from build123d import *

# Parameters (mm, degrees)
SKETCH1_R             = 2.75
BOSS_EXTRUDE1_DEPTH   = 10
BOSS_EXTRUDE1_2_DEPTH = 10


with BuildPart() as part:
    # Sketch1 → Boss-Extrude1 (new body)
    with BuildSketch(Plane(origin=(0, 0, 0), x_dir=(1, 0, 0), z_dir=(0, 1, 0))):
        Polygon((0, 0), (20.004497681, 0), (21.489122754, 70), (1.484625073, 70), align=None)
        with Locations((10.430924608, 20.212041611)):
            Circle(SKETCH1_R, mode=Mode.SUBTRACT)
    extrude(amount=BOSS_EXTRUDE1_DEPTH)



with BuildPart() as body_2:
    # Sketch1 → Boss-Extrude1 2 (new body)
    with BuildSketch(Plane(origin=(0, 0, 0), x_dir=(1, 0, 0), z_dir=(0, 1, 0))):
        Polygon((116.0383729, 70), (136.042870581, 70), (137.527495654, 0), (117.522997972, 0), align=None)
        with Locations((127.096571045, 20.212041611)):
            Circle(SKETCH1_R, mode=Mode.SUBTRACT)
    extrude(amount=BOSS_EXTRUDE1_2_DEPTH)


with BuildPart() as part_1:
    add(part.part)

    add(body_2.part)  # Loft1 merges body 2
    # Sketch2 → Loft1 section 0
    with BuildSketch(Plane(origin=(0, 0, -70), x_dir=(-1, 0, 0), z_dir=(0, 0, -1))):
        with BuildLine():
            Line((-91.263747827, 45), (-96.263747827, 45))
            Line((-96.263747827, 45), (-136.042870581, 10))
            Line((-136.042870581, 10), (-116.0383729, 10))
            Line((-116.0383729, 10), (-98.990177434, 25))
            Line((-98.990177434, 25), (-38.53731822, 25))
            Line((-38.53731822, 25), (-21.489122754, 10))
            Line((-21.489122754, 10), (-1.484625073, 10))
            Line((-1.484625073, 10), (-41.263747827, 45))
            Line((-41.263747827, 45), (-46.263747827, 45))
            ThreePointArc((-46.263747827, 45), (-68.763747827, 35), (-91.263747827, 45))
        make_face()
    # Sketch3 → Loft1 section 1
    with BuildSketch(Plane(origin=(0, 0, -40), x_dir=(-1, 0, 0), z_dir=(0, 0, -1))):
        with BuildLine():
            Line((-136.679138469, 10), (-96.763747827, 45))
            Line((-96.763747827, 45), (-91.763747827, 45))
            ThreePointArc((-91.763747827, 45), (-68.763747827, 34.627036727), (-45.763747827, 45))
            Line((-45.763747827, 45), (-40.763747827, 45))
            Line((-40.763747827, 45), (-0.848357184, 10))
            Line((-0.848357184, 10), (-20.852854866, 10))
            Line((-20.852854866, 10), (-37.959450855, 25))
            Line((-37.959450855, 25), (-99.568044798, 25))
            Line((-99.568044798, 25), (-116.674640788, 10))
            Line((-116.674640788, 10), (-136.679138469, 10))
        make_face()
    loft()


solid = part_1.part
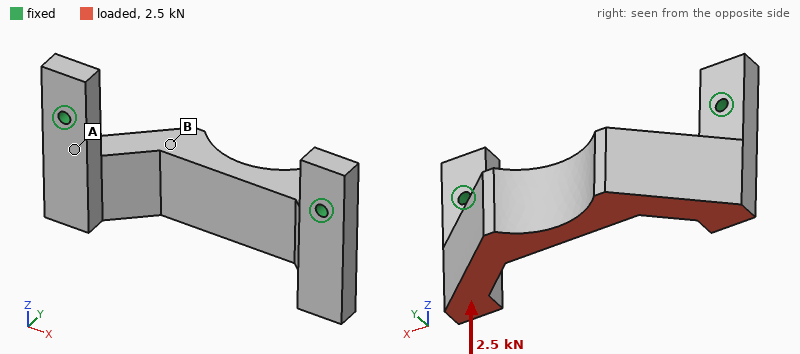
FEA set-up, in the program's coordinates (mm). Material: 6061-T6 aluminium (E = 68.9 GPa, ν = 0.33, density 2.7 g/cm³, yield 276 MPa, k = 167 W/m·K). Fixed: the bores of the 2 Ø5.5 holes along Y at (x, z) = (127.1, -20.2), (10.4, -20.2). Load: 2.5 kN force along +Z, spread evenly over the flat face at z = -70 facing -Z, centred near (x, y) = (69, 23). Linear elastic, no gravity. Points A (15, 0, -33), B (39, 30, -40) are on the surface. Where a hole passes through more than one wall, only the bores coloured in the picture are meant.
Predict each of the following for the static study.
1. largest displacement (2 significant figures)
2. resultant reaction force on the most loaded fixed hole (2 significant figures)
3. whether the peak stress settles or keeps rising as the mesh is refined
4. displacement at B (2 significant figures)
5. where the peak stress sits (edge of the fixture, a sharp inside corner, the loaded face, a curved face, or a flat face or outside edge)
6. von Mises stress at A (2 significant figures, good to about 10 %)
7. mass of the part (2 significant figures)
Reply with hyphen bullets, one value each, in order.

- 0.31 mm
- 1.3 kN
- keeps rising
- 0.15 mm
- edge of the fixture
- 58 MPa
- 220 g
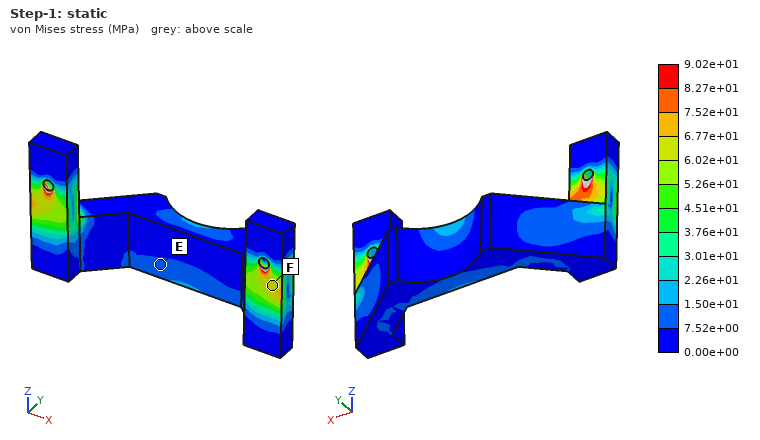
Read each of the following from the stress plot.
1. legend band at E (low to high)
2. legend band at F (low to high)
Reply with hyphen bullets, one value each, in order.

- 7.52e+00 to 1.50e+01 MPa
- 6.02e+01 to 6.77e+01 MPa
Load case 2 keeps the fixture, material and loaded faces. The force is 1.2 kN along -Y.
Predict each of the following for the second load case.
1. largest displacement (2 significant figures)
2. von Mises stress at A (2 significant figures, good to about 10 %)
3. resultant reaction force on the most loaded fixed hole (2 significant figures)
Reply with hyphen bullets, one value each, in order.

- 0.30 mm
- 64 MPa
- 650 N
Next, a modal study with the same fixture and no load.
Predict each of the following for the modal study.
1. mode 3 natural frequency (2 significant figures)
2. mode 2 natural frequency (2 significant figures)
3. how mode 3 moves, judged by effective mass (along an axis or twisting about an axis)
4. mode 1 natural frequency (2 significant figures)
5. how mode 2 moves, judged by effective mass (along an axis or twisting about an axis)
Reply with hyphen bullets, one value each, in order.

- 3100 Hz
- 2700 Hz
- along X
- 1000 Hz
- along X
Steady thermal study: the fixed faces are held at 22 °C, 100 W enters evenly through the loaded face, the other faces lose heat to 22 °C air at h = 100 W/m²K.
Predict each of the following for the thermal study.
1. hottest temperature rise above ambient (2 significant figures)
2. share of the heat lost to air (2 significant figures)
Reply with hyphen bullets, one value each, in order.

- 39 K
- 41 %
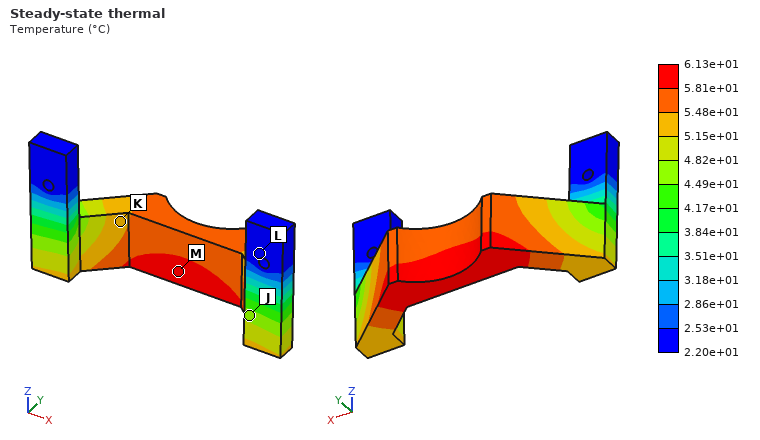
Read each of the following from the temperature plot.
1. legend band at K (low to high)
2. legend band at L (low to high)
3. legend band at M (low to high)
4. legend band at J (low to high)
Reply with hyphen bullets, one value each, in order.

- 5.15e+01 to 5.48e+01 °C
- 2.20e+01 to 2.53e+01 °C
- 5.81e+01 to 6.13e+01 °C
- 4.49e+01 to 4.82e+01 °C
